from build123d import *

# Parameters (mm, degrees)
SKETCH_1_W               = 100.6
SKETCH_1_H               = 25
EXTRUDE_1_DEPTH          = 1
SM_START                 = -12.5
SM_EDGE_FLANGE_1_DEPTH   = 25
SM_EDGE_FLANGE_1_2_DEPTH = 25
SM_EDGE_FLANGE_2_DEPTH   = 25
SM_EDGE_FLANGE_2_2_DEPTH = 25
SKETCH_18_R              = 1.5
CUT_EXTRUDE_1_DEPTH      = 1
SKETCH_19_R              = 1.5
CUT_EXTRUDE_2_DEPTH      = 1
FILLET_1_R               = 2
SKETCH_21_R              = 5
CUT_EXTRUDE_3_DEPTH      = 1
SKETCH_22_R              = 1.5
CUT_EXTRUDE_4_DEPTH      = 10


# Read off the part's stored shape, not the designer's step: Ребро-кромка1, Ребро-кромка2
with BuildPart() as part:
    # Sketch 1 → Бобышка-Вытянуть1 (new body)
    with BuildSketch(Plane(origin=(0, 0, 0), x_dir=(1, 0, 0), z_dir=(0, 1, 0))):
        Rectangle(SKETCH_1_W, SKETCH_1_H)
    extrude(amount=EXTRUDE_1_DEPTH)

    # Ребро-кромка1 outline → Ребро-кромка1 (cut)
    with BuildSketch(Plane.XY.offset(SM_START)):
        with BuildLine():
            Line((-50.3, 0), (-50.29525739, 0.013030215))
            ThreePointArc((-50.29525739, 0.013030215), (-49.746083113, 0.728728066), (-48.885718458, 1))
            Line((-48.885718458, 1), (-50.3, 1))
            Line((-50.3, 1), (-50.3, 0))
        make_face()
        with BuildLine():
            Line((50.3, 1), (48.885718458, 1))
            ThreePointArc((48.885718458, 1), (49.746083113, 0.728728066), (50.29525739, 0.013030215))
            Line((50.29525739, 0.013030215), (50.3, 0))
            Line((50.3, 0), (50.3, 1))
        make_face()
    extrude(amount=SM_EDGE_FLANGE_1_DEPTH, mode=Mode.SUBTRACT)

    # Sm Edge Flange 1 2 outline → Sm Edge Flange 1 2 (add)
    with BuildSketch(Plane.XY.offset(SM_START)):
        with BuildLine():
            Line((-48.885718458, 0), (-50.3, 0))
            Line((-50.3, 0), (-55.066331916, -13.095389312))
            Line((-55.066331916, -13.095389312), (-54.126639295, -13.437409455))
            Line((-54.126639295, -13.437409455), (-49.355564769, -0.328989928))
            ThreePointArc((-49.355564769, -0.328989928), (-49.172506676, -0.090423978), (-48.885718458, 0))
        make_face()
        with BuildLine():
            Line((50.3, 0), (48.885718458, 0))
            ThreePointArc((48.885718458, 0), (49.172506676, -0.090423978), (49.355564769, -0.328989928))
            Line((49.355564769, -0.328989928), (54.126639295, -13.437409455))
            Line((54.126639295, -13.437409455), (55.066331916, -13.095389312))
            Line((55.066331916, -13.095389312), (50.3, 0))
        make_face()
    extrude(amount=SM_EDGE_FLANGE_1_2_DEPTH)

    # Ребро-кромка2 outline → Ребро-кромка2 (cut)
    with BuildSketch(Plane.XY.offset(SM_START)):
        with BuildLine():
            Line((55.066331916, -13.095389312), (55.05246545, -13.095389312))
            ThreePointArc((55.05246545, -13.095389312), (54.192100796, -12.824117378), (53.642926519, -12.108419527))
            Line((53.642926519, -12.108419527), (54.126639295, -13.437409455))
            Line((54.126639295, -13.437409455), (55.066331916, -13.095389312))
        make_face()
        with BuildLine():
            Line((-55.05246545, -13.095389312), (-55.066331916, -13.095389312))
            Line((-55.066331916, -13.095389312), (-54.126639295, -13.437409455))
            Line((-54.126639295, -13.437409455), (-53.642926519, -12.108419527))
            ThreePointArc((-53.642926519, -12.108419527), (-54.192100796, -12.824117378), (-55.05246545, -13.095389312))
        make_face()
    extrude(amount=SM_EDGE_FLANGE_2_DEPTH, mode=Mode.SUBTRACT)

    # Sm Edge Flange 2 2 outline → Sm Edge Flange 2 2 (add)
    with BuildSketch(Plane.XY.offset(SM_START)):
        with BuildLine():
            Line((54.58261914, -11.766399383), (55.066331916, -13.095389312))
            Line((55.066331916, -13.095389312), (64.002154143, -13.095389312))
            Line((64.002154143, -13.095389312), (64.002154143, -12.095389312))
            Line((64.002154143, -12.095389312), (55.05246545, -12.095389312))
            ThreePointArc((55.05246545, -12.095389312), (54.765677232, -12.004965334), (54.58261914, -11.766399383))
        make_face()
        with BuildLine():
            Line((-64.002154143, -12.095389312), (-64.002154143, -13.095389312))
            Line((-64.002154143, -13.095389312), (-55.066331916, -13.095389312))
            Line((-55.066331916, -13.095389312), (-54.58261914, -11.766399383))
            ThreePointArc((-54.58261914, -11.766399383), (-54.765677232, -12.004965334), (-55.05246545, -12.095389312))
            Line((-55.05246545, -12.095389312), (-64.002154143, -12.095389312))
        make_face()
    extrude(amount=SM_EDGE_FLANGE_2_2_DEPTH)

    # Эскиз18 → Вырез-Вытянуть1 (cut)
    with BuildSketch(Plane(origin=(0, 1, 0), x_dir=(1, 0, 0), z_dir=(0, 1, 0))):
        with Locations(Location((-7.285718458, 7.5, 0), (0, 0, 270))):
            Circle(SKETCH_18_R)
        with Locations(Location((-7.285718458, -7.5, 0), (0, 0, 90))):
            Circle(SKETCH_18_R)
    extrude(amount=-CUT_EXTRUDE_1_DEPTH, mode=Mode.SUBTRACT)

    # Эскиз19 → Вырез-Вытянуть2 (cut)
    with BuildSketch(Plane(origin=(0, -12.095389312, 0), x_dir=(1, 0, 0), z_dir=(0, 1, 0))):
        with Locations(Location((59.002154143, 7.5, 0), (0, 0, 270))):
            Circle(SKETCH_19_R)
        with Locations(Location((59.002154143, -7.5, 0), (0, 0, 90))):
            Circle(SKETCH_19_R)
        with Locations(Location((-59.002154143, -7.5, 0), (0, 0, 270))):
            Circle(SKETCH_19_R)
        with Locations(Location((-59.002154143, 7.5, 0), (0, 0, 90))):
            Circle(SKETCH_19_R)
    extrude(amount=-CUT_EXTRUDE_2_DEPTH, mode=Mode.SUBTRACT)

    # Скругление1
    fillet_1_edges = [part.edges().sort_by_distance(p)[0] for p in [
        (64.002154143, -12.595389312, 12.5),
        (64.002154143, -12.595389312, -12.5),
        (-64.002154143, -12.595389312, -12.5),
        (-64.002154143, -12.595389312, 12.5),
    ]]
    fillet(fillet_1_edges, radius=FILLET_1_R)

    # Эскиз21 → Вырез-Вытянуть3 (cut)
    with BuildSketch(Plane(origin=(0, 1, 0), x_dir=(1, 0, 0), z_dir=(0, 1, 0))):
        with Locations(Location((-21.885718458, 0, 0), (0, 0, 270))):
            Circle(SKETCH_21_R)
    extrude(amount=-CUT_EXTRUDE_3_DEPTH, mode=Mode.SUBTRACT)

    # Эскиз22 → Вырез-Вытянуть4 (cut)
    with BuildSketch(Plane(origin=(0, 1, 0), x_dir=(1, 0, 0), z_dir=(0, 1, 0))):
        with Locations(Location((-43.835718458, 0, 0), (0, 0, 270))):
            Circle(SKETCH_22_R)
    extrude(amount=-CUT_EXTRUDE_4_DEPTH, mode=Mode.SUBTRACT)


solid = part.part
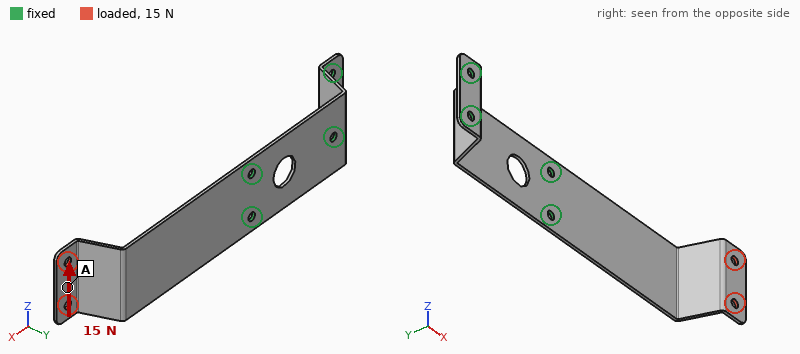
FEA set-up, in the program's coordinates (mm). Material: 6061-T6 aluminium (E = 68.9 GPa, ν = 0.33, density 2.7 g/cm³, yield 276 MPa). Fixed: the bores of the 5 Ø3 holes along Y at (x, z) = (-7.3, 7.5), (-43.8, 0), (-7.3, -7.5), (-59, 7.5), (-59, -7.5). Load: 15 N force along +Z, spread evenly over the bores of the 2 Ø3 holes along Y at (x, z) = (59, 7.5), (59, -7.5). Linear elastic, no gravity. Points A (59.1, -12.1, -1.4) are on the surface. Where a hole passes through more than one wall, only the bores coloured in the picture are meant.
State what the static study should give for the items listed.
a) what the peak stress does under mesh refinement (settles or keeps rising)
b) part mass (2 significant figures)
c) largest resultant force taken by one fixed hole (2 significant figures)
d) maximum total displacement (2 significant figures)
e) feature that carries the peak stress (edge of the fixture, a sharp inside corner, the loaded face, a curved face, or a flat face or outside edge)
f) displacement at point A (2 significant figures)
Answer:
keeps rising
9.5 g
57 N
0.80 mm
edge of the fixture
0.56 mm
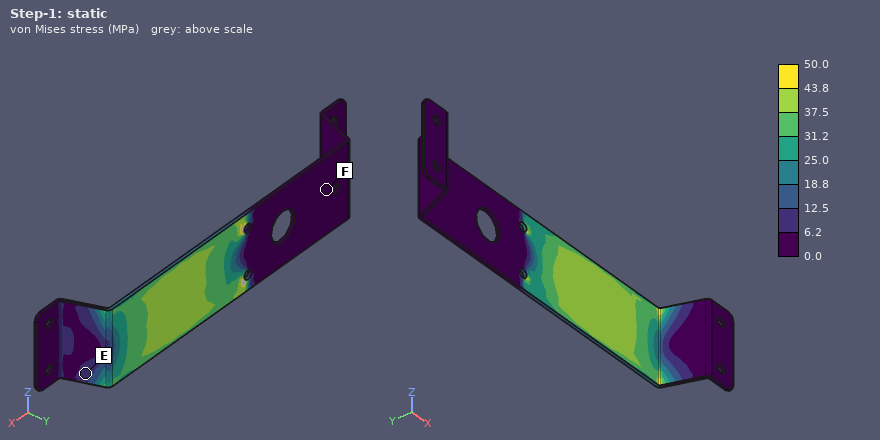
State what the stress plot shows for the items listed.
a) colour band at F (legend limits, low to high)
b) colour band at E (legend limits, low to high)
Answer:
0.0 to 6.2 MPa
6.2 to 12.5 MPa
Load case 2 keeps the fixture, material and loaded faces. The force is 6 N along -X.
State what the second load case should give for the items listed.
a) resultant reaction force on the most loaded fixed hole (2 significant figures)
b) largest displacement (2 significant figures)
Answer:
2.9 N
1.4 mm
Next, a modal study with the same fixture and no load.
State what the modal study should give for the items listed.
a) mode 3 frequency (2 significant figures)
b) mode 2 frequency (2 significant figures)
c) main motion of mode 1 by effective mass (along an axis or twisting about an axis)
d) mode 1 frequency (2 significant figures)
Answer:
820 Hz
610 Hz
along Y
150 Hz
